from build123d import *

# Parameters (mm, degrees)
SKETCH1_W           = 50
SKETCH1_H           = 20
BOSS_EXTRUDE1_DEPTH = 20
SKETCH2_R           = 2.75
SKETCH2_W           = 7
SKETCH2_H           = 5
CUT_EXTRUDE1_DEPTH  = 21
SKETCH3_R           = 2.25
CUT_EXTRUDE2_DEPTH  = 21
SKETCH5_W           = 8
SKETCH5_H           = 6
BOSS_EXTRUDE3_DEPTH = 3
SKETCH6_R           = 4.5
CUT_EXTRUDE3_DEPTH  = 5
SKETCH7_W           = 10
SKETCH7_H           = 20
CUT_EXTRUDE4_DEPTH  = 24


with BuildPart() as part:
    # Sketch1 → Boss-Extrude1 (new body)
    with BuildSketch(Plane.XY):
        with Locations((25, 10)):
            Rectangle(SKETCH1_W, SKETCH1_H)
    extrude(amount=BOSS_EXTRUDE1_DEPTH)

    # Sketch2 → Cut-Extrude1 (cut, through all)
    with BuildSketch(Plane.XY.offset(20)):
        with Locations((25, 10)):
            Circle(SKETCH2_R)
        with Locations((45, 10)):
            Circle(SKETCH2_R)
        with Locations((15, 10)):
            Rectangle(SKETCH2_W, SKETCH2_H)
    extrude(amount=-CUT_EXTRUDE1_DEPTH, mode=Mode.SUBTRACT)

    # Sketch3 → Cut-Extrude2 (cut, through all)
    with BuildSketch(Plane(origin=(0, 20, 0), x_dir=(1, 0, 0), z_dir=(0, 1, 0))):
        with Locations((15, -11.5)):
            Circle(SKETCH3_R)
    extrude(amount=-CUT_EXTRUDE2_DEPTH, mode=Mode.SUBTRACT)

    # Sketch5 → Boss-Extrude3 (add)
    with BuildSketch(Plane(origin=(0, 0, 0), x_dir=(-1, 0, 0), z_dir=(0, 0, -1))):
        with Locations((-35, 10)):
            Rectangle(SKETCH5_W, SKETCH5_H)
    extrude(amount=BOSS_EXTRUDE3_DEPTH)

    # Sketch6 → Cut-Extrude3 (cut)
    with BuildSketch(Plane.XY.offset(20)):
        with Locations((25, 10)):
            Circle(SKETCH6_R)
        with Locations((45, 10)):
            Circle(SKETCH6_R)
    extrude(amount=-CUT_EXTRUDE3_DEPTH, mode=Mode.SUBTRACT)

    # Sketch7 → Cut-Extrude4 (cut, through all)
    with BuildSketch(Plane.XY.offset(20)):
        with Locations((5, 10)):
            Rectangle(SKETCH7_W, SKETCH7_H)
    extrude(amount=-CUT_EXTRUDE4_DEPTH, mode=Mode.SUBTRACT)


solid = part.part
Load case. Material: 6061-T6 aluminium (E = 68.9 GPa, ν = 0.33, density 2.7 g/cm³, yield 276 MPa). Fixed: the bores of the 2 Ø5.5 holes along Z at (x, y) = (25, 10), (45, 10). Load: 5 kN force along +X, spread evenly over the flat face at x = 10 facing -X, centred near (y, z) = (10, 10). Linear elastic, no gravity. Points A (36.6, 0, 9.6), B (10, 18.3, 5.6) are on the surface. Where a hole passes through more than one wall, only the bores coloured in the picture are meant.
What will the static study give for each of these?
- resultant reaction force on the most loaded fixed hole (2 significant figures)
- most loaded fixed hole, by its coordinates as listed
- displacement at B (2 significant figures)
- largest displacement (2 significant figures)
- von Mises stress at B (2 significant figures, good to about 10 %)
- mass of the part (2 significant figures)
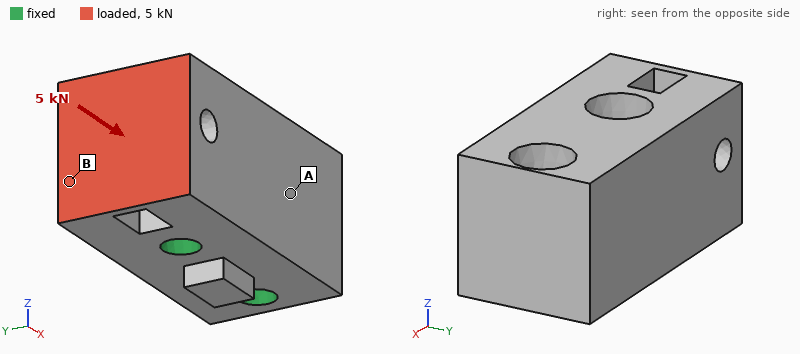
3.9 kN
(25, 10)
4.5 µm
12 µm
18 MPa
37 g
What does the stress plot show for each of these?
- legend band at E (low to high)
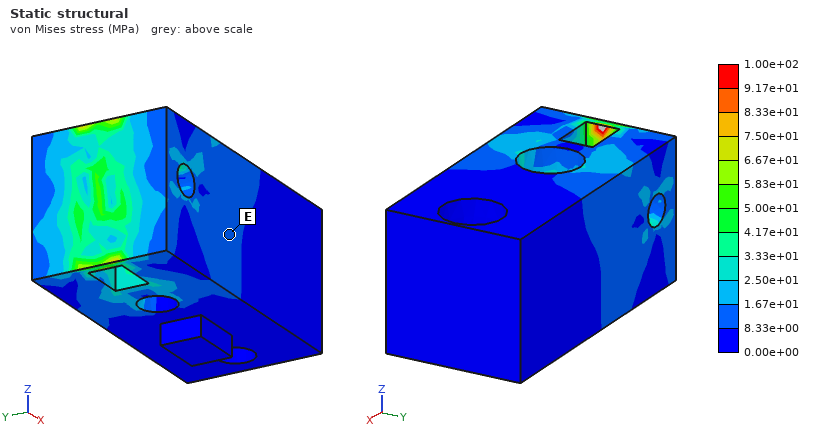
8.33e+00 to 1.67e+01 MPa
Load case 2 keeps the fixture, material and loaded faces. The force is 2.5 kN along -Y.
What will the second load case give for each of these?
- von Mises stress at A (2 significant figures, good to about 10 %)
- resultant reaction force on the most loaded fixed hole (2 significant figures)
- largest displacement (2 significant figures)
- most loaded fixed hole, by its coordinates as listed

8.4 MPa
3.7 kN
26 µm
(25, 10)
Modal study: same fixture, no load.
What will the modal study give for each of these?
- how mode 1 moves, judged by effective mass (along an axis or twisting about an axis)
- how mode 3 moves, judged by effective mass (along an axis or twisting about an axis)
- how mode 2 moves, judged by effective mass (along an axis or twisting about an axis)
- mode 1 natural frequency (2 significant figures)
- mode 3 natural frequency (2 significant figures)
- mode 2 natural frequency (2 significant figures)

along Y
twisting about X
along Z
27 kHz
34 kHz
31 kHz
